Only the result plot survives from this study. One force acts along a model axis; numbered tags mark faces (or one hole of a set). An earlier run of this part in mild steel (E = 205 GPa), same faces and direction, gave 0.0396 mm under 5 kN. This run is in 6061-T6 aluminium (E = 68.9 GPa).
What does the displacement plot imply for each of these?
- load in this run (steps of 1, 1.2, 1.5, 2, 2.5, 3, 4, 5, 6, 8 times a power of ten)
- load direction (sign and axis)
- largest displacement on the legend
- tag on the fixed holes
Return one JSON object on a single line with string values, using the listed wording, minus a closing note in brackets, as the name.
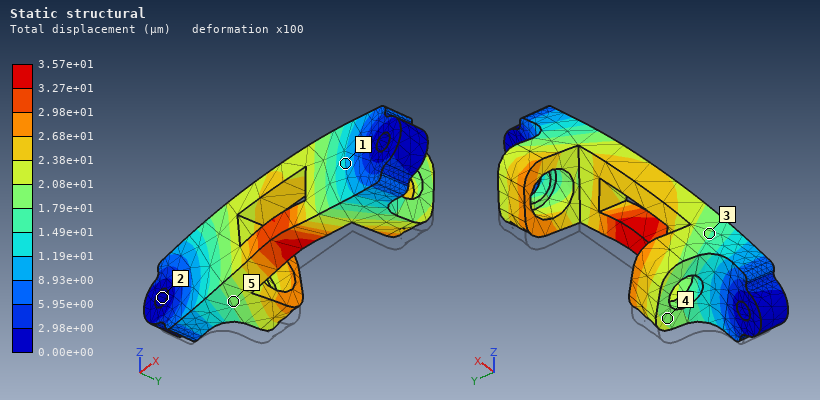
{"load in this run": "1.5 kN", "load direction": "+Z", "largest displacement on the legend": "3.57e+01 µm", "tag on the fixed holes": "2"}
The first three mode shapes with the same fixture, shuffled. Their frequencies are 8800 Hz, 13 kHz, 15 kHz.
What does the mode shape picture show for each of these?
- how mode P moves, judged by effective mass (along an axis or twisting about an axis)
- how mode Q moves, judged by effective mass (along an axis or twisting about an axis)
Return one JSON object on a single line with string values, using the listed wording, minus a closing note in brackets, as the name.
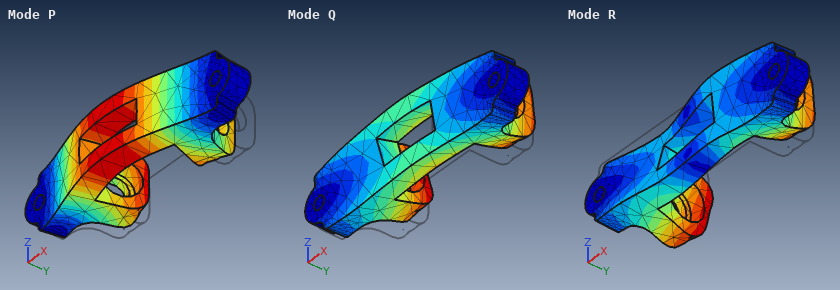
{"how mode P moves, judged by effective mass": "along Y", "how mode Q moves, judged by effective mass": "along Z"}
